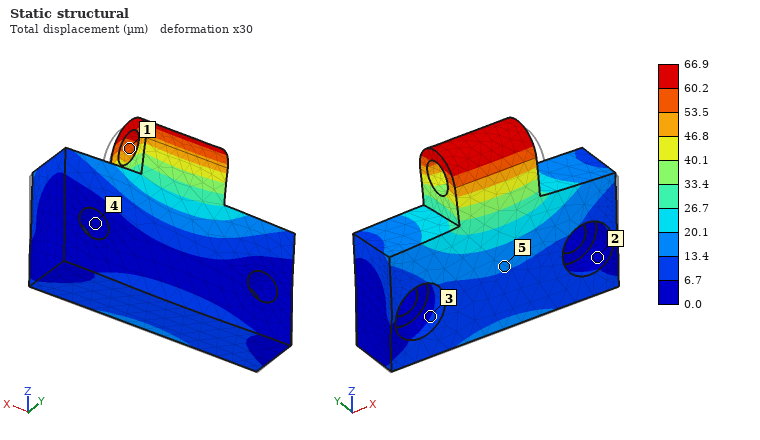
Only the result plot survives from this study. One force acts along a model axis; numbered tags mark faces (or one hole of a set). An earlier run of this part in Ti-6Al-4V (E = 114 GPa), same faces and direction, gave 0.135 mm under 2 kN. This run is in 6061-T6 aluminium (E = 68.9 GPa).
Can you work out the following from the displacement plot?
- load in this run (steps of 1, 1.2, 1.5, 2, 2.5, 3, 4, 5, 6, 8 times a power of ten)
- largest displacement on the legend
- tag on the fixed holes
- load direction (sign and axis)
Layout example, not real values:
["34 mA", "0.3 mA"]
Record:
["600 N", "66.9 µm", "4", "+Y"]
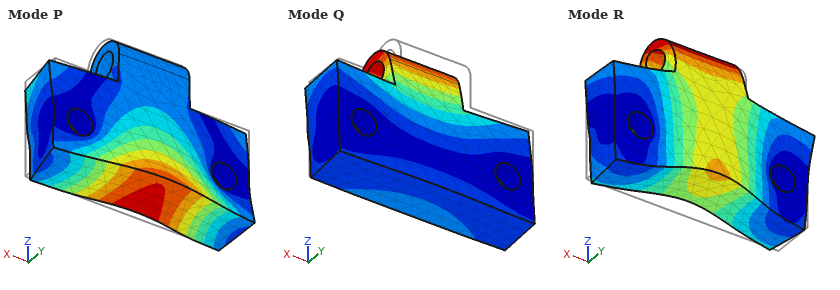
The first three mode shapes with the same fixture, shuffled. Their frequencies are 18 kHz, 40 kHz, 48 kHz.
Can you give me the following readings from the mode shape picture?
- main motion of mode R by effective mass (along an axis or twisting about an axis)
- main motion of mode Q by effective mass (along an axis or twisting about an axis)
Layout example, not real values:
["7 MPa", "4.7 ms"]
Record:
["along Z", "along Y"]
